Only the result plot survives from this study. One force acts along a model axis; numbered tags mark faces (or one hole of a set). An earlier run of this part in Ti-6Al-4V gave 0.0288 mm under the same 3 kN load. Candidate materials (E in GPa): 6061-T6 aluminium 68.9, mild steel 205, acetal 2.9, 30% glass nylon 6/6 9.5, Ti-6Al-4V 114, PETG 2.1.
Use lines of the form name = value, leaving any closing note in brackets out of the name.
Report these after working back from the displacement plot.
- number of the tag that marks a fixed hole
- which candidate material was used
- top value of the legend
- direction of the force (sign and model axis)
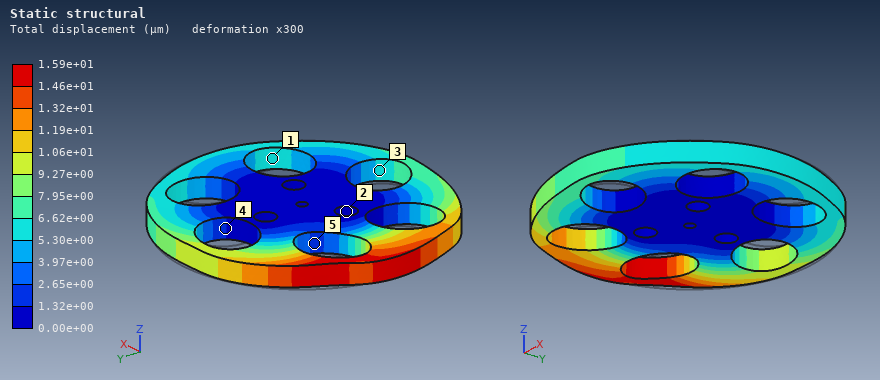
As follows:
number of the tag that marks a fixed hole = 2
which candidate material was used = mild steel
top value of the legend = 1.59e+01 µm
direction of the force = -Y
